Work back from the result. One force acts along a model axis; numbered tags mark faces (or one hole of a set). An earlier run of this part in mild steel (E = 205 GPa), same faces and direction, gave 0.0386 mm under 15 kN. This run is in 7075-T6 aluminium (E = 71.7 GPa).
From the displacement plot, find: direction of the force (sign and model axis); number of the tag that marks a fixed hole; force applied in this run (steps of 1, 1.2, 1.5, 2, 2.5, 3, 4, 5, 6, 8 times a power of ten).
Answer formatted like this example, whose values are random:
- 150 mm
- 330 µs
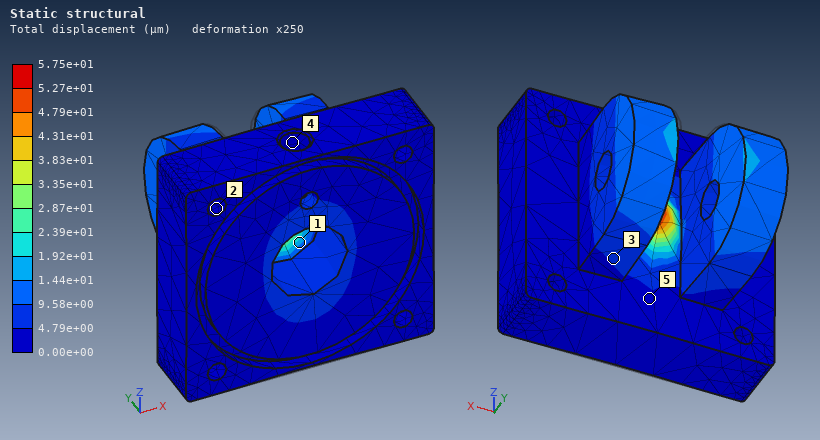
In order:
- +Y
- 2
- 8 kN
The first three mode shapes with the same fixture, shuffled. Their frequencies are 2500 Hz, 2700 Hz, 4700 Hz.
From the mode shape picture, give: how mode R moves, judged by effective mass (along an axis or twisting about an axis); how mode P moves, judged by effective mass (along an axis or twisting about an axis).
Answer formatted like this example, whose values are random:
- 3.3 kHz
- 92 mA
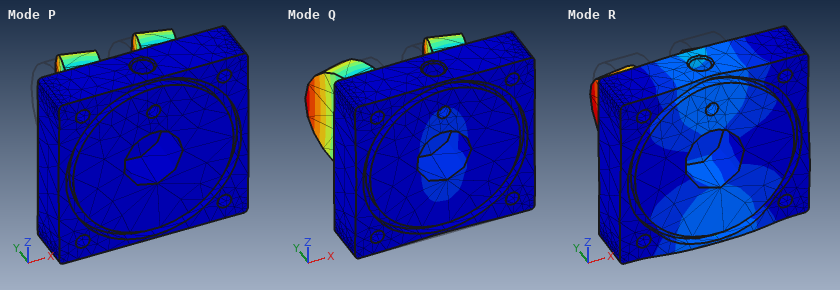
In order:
- along Z
- along X
